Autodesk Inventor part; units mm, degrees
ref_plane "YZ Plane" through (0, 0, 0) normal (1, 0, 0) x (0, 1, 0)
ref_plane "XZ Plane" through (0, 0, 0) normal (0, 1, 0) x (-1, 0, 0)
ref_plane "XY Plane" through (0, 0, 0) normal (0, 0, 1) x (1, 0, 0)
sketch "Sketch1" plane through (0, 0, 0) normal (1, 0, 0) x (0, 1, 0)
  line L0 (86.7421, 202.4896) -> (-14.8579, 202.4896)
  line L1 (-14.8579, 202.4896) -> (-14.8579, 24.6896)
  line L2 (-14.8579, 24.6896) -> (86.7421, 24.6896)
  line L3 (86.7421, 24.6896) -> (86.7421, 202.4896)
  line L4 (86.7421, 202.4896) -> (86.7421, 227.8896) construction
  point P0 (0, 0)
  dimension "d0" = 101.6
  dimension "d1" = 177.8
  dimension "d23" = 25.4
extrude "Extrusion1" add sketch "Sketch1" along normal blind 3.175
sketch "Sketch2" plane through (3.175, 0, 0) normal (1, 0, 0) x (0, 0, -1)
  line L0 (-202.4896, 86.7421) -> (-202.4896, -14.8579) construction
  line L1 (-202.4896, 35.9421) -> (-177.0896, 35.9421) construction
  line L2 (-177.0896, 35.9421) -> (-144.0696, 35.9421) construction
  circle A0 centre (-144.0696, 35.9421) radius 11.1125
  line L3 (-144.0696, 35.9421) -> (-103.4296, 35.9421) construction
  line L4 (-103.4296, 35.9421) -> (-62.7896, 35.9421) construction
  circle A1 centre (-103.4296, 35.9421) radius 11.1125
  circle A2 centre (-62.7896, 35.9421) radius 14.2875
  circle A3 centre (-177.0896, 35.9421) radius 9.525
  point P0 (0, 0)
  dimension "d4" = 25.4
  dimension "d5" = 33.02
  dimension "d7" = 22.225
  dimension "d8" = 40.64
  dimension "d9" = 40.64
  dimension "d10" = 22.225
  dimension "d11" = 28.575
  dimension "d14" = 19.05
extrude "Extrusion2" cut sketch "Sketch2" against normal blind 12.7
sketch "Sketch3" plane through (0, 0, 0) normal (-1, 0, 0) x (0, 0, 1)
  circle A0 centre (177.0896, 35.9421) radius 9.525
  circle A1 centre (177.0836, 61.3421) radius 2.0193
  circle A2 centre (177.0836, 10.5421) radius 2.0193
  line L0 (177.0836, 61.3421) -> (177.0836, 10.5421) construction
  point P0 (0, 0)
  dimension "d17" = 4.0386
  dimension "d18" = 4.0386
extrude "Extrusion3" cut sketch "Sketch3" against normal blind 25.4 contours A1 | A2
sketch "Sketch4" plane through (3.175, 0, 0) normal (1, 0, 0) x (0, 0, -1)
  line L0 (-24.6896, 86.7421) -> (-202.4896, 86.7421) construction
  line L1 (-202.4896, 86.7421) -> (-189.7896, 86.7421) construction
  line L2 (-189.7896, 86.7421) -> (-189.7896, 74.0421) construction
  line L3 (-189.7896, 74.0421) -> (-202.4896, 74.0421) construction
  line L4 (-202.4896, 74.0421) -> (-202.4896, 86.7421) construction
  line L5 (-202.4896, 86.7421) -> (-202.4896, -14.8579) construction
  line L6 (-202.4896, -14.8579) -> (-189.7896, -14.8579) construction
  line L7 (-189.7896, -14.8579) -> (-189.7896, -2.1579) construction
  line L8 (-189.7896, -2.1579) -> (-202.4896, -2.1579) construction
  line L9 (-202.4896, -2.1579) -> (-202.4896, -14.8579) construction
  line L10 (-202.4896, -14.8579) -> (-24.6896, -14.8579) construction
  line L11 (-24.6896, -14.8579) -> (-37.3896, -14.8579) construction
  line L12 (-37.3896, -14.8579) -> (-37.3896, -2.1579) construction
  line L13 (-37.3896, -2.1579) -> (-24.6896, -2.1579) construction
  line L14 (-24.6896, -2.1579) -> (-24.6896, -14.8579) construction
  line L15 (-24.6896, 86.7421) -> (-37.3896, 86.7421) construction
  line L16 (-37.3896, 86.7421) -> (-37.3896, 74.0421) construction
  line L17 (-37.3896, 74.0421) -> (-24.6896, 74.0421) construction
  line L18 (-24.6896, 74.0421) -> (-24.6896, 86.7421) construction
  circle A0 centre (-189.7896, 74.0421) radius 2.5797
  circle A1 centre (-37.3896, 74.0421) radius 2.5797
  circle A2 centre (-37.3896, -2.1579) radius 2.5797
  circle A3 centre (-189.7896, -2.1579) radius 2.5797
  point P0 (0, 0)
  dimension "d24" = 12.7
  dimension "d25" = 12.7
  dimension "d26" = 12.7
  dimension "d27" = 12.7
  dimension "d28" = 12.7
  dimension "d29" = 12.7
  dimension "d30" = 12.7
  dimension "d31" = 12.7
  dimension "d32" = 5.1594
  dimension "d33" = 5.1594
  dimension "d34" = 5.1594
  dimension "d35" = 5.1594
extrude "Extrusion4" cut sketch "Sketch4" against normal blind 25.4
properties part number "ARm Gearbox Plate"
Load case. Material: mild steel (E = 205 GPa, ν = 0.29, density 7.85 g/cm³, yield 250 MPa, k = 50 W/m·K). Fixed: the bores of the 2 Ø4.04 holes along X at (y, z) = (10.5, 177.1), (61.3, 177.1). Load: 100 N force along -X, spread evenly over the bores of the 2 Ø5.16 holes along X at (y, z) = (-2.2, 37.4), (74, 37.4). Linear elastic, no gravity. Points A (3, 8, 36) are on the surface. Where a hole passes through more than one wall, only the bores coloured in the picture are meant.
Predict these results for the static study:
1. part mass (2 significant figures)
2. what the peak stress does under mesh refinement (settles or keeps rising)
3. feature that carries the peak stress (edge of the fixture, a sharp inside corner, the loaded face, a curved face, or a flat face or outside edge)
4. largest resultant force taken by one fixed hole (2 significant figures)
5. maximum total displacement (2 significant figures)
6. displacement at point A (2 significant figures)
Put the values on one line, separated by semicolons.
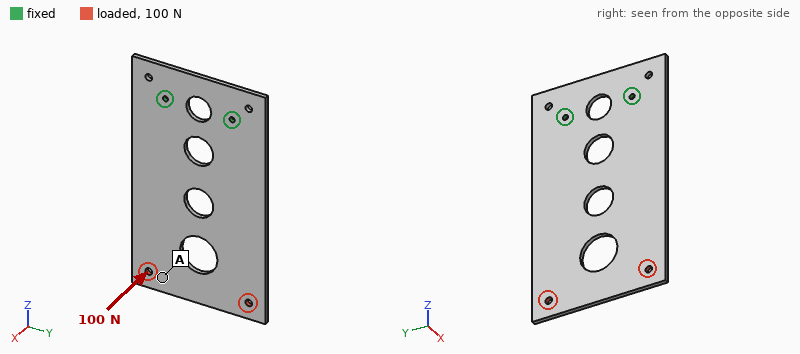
410 g; keeps rising; edge of the fixture; 50 N; 2.3 mm; 2.0 mm
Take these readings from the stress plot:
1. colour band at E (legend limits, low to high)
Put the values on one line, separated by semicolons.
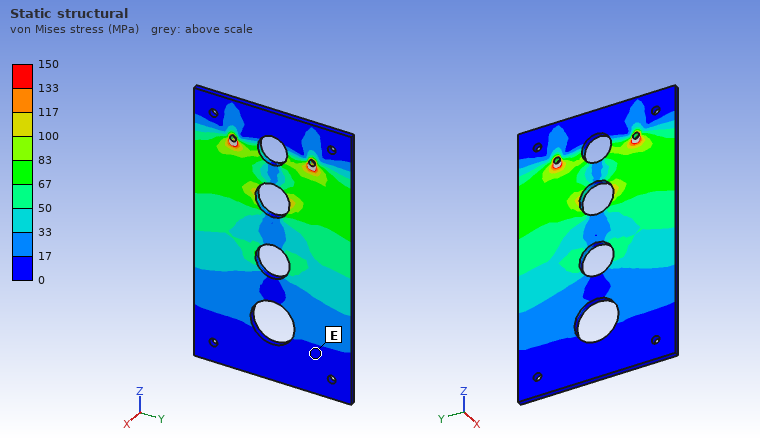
0 to 17 MPa
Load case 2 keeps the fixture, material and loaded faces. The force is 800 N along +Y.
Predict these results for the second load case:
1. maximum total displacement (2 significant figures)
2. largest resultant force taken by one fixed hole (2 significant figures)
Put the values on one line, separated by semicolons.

44 µm; 2.1 kN
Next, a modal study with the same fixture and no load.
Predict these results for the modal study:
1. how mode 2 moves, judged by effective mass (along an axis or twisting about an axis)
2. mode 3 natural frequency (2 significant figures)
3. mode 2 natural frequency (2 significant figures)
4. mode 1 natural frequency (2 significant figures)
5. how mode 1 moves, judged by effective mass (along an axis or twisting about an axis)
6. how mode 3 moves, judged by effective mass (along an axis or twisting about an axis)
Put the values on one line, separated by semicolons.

twisting about Z; 650 Hz; 350 Hz; 110 Hz; along X; along X
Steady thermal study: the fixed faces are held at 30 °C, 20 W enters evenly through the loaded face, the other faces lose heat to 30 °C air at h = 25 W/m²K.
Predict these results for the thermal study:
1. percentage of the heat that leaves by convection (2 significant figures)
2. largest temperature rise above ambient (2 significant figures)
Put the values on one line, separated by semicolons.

91 %; 79 K
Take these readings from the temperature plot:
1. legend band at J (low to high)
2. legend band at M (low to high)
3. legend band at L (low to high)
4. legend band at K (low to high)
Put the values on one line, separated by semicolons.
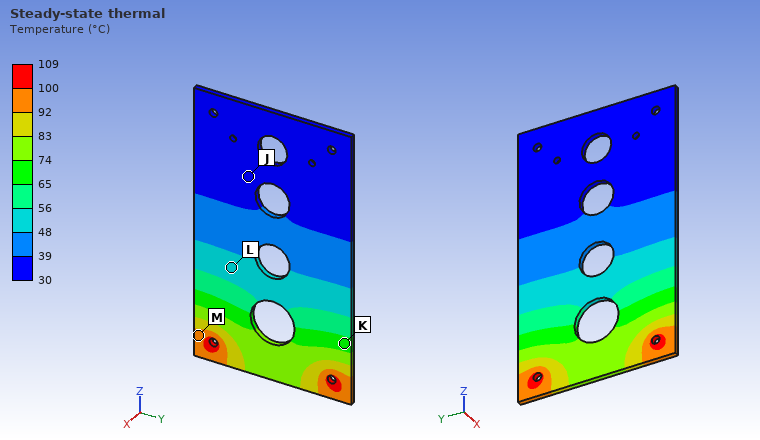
30 to 39 °C; 92 to 100 °C; 48 to 56 °C; 65 to 74 °C
